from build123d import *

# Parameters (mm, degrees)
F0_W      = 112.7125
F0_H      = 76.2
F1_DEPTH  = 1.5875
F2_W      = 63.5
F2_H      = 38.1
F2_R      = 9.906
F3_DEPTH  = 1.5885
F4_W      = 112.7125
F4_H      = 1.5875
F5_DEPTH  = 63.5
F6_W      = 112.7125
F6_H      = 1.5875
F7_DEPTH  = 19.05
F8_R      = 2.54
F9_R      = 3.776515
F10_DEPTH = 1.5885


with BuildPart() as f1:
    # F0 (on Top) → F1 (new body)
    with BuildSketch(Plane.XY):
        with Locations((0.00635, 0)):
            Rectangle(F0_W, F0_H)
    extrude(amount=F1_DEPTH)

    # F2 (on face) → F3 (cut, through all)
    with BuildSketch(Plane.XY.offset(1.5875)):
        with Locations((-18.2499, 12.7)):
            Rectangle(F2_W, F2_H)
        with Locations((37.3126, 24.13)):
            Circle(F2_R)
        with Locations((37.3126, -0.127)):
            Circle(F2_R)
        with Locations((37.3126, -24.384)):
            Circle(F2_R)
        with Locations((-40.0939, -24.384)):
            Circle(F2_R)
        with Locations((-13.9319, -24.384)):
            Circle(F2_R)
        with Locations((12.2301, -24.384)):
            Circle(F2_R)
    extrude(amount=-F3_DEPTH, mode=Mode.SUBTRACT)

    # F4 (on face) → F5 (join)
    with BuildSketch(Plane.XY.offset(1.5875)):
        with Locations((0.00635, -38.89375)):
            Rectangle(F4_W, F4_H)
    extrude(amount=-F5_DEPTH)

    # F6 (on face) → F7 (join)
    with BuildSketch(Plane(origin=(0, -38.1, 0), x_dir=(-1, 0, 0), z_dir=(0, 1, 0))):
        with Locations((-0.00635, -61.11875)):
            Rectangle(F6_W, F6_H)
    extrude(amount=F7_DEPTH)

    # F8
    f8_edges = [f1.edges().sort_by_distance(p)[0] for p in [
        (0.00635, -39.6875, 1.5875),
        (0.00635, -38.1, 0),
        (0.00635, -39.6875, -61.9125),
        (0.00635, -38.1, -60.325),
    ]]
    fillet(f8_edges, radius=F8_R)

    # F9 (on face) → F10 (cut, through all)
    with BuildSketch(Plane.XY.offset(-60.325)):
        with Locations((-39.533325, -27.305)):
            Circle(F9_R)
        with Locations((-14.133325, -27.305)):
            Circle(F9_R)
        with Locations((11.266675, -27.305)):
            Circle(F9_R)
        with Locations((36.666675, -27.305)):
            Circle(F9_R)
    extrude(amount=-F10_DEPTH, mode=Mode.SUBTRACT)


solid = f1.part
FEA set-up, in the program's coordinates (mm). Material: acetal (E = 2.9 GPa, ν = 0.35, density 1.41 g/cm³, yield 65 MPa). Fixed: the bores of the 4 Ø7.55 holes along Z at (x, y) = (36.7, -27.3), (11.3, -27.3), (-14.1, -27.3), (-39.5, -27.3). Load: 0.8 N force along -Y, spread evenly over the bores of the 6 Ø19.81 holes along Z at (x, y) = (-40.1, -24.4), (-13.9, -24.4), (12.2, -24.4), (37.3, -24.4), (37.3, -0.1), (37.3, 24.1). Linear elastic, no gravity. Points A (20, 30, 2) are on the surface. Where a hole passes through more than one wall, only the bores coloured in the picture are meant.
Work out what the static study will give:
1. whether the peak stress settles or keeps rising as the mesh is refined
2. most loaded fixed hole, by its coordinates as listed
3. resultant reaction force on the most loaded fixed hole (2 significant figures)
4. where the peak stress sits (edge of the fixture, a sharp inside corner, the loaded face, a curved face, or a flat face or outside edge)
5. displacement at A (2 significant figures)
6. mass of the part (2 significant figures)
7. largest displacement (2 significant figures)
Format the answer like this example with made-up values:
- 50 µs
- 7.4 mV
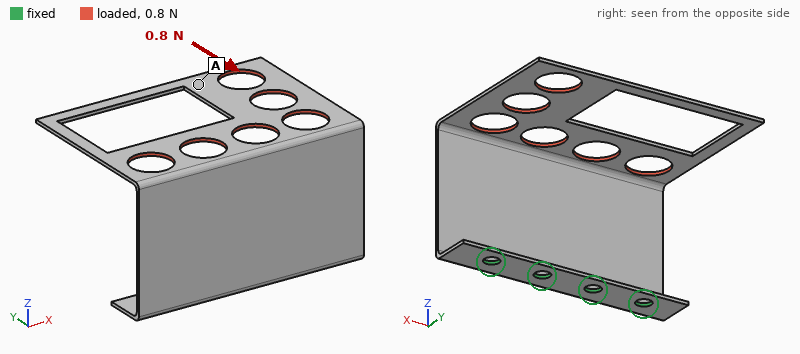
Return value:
- keeps rising
- (36.7, -27.3)
- 0.32 N
- edge of the fixture
- 1.3 mm
- 30 g
- 1.5 mm
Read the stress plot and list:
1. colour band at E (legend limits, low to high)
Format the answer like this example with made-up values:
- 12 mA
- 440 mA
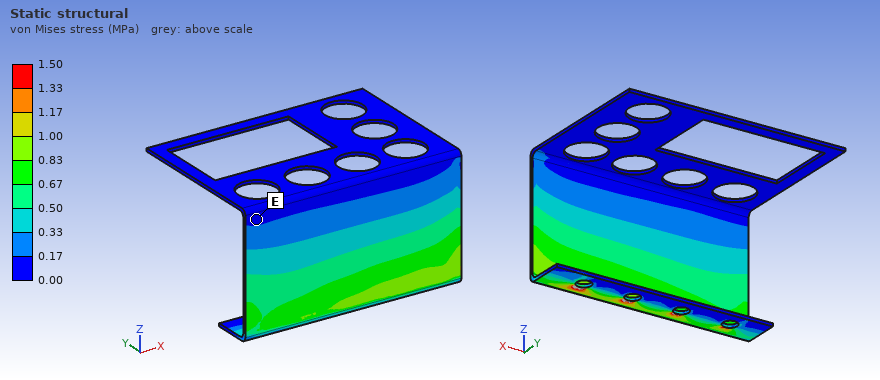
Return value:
- 0.00 to 0.17 MPa
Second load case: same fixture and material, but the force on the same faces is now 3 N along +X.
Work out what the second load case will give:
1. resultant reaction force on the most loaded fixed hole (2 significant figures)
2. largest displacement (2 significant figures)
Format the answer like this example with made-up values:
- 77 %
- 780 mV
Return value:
- 2.4 N
- 1.8 mm
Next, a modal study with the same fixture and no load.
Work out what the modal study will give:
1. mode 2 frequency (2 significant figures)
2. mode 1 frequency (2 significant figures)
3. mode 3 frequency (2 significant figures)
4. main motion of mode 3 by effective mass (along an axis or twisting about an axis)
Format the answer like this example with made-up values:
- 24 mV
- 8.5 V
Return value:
- 56 Hz
- 32 Hz
- 67 Hz
- along Y
